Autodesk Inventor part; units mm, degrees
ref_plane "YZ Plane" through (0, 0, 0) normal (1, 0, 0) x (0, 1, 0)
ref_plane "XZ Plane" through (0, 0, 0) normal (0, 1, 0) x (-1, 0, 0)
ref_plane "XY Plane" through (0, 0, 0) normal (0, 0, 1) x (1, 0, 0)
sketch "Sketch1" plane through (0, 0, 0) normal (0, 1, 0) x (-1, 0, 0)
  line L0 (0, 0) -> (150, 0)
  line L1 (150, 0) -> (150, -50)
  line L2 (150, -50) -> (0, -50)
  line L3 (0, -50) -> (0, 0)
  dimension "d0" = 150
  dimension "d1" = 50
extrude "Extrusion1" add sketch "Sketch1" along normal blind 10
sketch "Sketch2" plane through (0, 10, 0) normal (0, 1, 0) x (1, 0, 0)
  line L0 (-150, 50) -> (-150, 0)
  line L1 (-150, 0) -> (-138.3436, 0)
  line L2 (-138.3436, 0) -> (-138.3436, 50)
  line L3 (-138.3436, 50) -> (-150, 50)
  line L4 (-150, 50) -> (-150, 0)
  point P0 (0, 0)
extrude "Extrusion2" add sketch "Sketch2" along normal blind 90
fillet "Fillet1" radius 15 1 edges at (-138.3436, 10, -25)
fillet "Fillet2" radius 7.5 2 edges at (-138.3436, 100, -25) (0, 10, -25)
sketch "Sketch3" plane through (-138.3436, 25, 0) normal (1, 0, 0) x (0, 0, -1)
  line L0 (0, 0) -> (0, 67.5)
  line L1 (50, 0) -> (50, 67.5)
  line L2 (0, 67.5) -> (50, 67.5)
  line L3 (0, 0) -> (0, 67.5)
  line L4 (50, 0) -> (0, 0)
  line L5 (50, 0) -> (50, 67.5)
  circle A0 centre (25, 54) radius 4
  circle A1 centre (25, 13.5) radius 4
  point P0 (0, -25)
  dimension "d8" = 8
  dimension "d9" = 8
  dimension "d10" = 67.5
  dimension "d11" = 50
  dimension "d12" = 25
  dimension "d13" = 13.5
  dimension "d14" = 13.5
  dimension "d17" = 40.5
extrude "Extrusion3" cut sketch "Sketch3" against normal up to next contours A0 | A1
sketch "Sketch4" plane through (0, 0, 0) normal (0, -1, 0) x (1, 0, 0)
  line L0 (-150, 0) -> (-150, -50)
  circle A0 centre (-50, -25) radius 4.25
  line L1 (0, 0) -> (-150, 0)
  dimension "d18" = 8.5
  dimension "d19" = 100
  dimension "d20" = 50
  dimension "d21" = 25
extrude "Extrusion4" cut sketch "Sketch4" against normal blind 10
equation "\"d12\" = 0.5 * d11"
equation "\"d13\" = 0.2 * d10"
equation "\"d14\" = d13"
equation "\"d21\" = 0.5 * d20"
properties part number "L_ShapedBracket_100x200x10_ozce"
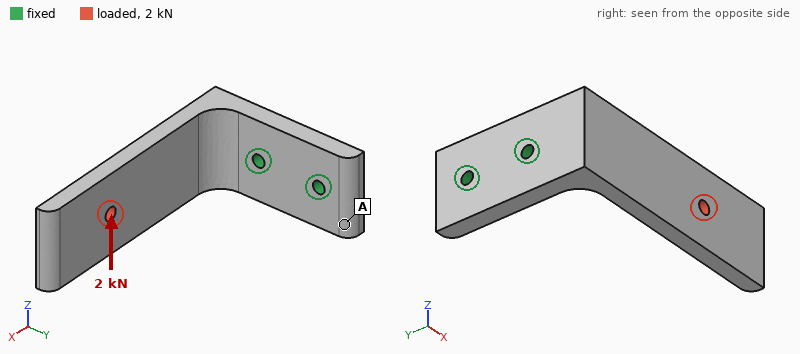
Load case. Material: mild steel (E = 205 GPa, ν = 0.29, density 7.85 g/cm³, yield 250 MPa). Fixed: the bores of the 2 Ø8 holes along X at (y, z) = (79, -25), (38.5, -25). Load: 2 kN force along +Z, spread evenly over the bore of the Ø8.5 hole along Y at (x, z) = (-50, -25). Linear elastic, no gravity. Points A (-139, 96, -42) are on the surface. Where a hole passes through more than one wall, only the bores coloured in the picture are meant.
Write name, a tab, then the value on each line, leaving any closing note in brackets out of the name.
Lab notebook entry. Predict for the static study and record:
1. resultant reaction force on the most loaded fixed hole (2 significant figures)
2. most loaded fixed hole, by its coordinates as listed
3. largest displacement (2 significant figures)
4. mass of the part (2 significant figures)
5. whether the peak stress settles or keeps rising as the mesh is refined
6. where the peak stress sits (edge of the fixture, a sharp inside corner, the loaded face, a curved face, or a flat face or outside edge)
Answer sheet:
resultant reaction force on the most loaded fixed hole	3.2 kN
most loaded fixed hole, by its coordinates as listed	(38.5, -25)
largest displacement	0.41 mm
mass of the part	1000 g
whether the peak stress settles or keeps rising as the mesh is refined	keeps rising
where the peak stress sits	edge of the fixture
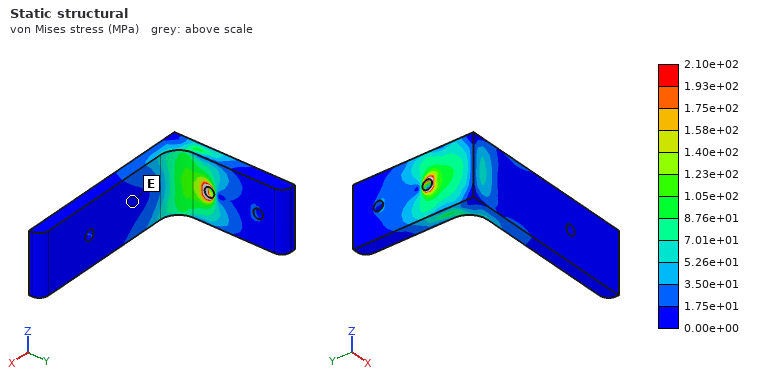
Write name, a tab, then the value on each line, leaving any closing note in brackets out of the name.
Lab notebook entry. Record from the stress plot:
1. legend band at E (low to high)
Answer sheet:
legend band at E	0.00e+00 to 1.75e+01 MPa
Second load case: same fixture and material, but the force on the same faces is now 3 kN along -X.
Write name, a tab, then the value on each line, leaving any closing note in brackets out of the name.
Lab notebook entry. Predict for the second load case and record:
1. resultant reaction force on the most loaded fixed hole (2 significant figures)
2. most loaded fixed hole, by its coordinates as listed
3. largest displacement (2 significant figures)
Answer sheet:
resultant reaction force on the most loaded fixed hole	3.8 kN
most loaded fixed hole, by its coordinates as listed	(38.5, -25)
largest displacement	0.19 mm
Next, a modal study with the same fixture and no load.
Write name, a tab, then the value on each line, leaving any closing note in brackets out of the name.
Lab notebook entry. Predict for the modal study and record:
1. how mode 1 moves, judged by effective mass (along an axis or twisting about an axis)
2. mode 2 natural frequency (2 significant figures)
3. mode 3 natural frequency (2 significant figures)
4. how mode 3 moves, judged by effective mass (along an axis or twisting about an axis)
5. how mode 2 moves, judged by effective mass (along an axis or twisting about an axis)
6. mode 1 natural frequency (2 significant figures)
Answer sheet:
how mode 1 moves, judged by effective mass	along Y
mode 2 natural frequency	660 Hz
mode 3 natural frequency	1800 Hz
how mode 3 moves, judged by effective mass	along X
how mode 2 moves, judged by effective mass	along Z
mode 1 natural frequency	370 Hz
